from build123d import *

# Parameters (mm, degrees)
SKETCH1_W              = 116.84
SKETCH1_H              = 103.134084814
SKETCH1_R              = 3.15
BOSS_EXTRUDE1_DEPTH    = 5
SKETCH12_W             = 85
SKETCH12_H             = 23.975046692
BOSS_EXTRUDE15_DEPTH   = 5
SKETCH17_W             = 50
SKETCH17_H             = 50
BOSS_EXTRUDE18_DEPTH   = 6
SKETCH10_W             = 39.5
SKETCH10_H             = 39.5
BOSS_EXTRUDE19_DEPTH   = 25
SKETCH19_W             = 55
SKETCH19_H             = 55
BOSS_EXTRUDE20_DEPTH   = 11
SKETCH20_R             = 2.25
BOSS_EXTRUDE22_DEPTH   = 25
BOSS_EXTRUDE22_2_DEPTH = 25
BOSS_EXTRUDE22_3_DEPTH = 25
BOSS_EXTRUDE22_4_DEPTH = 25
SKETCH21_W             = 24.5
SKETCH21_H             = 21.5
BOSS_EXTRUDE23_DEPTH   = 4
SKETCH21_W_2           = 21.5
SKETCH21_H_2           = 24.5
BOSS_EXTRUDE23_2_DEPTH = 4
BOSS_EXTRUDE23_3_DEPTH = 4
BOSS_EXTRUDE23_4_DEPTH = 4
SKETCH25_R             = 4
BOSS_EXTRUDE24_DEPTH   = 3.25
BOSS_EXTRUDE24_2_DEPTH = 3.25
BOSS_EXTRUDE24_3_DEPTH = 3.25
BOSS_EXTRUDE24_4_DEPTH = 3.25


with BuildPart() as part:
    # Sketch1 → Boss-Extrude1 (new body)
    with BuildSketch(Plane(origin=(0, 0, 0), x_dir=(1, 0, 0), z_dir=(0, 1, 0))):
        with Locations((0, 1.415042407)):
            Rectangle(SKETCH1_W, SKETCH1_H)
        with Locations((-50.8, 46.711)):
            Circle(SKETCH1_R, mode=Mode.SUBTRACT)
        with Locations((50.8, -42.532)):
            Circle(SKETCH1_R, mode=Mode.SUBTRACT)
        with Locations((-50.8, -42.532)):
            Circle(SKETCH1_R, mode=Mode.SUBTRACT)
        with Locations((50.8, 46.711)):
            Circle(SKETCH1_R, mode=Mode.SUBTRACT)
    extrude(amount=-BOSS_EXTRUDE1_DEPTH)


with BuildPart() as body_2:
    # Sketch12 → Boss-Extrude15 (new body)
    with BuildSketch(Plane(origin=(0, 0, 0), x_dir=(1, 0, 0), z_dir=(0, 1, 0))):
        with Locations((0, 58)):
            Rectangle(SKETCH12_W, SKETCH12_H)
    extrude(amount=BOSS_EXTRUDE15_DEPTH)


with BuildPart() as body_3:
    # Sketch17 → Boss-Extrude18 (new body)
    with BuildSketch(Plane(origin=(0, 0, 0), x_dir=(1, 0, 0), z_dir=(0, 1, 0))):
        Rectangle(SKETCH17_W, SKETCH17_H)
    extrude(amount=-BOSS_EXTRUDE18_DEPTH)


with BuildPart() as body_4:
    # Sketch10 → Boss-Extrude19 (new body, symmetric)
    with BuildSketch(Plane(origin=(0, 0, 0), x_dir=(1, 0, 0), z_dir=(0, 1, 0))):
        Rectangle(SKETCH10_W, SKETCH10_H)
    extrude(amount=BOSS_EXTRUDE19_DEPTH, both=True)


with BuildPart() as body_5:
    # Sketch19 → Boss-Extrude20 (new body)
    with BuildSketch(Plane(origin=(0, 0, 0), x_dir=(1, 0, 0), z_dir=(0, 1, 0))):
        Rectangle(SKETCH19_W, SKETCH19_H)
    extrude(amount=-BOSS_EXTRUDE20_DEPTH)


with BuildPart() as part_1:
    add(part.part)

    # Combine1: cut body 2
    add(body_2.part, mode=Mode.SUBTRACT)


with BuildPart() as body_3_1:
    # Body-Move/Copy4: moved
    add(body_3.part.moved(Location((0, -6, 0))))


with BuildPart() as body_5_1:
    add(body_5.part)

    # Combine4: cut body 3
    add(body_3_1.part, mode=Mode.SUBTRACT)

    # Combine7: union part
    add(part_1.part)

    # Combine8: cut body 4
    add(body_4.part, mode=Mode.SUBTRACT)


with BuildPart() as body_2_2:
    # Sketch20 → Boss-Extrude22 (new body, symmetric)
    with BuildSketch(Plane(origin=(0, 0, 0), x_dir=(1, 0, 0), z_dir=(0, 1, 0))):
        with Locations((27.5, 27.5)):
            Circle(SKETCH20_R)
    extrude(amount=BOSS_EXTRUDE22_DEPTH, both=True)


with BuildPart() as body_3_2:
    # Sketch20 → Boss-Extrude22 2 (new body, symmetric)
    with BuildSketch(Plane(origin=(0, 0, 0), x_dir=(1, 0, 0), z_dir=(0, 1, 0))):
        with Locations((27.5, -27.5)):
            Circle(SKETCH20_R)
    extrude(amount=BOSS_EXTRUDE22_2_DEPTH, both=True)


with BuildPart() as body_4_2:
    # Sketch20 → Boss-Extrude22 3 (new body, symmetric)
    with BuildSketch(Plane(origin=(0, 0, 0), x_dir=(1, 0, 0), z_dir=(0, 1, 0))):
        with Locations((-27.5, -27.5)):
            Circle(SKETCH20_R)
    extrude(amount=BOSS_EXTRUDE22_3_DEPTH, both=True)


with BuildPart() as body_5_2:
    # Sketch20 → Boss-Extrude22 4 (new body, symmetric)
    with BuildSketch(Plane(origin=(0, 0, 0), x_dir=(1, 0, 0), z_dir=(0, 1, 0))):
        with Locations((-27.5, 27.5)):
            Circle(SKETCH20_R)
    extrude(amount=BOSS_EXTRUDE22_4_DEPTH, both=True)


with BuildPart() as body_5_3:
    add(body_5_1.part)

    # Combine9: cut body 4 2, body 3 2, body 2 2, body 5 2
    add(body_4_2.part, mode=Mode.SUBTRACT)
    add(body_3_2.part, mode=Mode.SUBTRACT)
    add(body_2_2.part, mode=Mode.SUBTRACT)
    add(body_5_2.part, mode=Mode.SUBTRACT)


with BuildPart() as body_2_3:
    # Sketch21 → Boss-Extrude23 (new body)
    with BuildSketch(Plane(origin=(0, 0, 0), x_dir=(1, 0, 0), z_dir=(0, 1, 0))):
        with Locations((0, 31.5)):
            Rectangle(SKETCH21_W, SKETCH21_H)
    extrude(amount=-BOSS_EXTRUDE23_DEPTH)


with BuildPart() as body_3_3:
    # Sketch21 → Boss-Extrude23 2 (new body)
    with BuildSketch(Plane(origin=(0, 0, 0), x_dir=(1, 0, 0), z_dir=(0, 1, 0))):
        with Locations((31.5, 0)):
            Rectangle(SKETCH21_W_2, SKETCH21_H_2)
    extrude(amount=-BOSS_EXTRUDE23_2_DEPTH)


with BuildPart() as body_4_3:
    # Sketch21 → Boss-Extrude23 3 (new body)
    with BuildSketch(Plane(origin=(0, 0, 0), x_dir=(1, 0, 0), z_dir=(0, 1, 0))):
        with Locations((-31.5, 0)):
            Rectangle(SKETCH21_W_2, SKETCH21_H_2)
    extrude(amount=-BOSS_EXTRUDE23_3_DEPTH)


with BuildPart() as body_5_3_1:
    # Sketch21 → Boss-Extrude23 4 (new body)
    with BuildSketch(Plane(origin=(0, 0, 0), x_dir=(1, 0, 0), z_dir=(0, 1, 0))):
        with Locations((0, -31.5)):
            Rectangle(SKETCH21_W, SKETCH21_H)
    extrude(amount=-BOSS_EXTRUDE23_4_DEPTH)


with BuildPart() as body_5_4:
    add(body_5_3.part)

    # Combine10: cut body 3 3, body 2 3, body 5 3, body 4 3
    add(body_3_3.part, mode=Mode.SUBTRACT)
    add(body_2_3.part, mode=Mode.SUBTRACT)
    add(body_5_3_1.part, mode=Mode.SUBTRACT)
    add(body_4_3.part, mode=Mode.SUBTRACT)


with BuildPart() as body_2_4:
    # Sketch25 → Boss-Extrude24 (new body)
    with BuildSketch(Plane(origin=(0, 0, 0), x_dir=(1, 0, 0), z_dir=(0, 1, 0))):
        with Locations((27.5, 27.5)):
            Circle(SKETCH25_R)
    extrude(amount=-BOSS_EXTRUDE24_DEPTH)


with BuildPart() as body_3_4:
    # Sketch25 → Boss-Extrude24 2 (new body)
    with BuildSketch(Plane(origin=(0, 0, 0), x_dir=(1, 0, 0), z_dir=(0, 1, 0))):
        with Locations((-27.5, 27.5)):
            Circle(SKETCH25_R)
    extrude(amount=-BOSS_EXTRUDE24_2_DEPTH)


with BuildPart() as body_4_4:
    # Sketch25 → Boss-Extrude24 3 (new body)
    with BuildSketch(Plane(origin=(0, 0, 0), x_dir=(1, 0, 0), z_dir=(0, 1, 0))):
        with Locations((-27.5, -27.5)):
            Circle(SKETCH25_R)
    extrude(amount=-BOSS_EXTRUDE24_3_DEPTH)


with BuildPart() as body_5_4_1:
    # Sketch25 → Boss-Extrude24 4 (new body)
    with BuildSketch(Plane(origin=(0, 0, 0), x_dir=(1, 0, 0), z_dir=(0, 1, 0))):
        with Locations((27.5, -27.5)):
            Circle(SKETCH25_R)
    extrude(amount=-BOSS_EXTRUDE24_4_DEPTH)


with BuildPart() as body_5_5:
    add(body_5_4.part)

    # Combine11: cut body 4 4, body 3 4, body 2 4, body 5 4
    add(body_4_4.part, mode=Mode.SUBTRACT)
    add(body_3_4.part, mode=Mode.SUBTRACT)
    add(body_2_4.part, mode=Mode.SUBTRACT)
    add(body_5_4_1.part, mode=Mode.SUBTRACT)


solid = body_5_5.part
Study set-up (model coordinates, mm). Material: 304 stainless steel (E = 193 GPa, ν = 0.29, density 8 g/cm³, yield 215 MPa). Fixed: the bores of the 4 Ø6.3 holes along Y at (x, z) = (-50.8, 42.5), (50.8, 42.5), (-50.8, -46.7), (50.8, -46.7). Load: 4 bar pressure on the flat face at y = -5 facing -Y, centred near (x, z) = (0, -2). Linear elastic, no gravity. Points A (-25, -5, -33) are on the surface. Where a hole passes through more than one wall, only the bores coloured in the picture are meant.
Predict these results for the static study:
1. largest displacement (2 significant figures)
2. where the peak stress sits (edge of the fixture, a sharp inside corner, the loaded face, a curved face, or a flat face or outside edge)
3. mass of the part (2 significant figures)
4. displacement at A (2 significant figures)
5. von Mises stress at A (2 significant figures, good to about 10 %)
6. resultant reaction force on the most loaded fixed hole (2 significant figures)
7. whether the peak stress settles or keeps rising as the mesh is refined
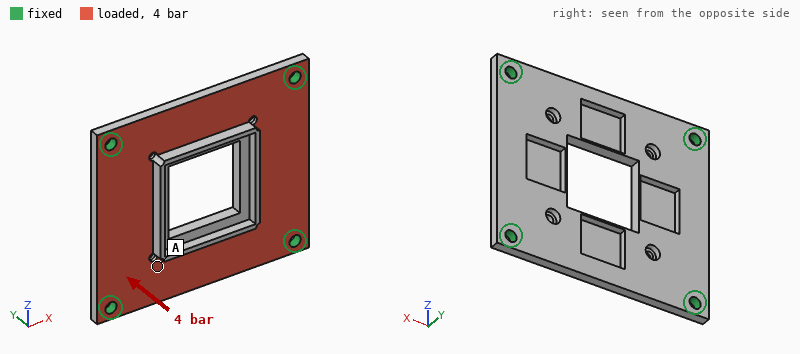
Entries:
63 µm
edge of the fixture
370 g
42 µm
29 MPa
1.1 kN
keeps rising
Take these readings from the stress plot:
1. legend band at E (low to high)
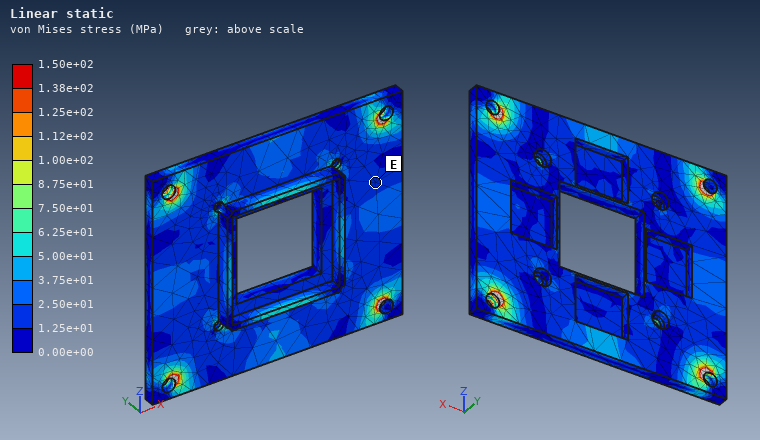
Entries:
1.25e+01 to 2.50e+01 MPa
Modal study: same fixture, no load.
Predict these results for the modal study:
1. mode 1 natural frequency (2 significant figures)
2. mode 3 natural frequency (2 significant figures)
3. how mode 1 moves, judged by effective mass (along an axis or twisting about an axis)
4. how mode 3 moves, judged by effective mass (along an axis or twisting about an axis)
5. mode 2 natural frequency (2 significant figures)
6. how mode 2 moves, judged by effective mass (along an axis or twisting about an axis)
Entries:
2300 Hz
3400 Hz
along Y
twisting about Z
3000 Hz
twisting about X
